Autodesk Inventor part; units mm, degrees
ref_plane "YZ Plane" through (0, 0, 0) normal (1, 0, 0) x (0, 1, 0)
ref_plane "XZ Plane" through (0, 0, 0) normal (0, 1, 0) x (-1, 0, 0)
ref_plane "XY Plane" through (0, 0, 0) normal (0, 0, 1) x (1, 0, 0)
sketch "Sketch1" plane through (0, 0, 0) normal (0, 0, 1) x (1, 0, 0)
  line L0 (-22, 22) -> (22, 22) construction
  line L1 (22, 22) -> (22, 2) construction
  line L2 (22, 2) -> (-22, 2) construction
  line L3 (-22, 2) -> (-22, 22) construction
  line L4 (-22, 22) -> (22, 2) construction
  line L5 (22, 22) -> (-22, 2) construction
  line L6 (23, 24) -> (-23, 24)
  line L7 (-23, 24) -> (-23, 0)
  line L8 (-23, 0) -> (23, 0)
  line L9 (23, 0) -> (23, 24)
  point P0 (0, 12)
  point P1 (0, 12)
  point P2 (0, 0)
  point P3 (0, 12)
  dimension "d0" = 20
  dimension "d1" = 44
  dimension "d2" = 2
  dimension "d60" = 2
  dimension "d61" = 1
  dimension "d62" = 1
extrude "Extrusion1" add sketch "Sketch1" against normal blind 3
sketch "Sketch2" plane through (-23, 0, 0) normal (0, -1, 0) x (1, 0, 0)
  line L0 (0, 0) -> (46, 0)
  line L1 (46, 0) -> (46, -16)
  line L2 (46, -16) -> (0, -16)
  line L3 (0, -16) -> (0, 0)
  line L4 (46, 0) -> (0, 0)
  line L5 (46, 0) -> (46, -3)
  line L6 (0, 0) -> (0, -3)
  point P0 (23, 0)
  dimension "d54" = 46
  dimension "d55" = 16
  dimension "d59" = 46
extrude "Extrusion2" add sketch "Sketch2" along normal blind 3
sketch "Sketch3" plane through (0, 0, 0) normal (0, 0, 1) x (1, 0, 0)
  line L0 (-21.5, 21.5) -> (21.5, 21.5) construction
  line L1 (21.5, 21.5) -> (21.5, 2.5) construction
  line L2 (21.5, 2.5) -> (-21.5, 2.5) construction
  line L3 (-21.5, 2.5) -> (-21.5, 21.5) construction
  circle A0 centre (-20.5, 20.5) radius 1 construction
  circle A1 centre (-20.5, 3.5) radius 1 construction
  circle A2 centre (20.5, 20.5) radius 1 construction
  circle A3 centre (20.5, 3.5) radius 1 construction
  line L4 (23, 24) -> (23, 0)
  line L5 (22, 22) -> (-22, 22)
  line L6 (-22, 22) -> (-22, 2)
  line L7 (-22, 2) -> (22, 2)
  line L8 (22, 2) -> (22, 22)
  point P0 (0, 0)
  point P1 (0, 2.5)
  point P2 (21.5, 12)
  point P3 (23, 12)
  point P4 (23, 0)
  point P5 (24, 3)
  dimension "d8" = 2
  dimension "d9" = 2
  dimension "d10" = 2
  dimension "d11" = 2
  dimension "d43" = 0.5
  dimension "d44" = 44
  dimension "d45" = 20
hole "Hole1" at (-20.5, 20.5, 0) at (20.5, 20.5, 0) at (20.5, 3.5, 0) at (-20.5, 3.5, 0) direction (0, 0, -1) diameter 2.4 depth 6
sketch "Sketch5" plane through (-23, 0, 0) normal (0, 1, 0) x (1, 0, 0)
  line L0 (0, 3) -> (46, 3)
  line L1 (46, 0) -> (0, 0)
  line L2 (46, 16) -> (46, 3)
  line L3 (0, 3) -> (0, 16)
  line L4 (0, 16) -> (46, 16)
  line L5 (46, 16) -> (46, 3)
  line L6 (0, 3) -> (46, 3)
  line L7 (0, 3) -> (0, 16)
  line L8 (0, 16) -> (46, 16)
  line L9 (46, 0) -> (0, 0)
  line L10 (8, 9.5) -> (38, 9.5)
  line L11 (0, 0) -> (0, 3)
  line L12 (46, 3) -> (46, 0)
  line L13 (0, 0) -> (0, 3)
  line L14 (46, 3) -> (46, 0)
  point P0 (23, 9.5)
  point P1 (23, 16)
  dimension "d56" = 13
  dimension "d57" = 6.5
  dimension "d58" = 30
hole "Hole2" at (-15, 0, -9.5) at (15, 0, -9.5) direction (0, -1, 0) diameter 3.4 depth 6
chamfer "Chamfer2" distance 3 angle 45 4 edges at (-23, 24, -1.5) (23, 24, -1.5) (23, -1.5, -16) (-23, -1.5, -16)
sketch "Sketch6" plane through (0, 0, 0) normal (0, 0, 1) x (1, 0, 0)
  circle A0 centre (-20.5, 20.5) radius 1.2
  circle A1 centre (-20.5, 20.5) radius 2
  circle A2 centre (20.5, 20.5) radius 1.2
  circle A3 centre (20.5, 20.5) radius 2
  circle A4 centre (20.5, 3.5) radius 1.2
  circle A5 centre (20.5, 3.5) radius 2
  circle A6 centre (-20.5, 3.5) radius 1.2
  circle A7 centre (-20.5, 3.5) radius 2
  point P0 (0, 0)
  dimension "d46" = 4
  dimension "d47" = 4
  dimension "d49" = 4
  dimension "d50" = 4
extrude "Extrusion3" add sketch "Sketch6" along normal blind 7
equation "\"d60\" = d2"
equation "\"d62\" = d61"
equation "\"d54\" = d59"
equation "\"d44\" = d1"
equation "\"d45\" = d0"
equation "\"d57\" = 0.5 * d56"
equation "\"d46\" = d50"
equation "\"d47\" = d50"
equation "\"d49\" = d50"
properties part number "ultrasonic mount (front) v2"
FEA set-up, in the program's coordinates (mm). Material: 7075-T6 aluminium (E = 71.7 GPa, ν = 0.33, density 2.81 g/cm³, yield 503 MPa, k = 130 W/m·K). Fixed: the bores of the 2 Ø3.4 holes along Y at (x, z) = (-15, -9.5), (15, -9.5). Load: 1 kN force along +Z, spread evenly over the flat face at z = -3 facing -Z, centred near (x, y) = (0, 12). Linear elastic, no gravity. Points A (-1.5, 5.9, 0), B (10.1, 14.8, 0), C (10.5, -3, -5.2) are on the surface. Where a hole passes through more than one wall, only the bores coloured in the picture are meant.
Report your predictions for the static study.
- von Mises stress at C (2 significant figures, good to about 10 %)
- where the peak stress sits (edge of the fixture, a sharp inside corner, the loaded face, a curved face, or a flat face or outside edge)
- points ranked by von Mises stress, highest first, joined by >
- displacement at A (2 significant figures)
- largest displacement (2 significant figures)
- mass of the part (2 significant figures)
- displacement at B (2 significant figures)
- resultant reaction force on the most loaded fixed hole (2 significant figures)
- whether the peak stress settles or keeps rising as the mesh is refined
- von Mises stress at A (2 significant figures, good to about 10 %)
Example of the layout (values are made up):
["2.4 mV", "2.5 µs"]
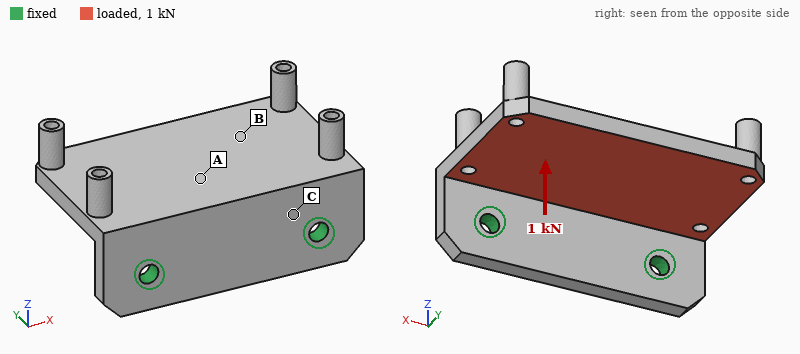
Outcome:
["170 MPa", "edge of the fixture", "C > A > B", "0.18 mm", "0.66 mm", "16 g", "0.39 mm", "510 N", "keeps rising", "88 MPa"]
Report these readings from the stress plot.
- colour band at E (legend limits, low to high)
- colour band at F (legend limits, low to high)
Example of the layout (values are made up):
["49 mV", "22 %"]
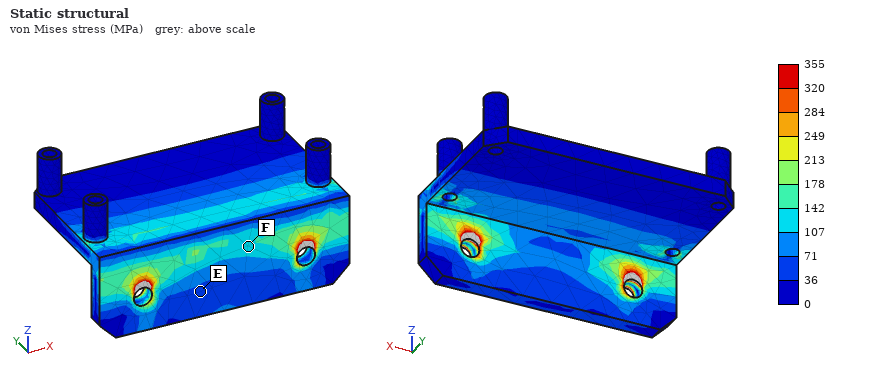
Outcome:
["36 to 71 MPa", "107 to 142 MPa"]
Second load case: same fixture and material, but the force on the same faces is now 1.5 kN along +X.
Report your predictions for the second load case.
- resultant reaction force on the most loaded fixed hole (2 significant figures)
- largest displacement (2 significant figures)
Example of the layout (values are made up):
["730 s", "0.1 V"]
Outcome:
["1.0 kN", "0.12 mm"]
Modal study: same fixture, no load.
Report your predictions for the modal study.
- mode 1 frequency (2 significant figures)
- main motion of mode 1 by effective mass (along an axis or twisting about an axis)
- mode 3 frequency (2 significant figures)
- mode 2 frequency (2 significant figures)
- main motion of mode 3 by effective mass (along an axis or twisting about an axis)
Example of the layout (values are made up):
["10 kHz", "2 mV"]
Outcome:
["2400 Hz", "along Z", "8700 Hz", "4600 Hz", "along X"]
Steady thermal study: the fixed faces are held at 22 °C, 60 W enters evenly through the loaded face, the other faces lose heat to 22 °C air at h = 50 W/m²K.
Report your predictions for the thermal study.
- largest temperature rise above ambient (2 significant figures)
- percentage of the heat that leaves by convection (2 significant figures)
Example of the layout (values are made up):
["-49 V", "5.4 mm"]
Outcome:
["71 K", "12 %"]
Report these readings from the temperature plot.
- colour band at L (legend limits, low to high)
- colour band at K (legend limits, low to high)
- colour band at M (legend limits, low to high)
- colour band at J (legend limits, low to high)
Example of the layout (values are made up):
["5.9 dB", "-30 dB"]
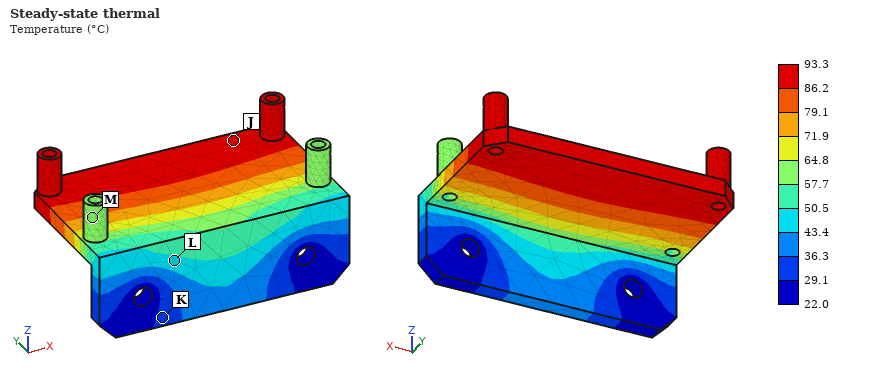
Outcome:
["43.4 to 50.5 °C", "29.1 to 36.3 °C", "57.7 to 64.8 °C", "86.2 to 93.3 °C"]
